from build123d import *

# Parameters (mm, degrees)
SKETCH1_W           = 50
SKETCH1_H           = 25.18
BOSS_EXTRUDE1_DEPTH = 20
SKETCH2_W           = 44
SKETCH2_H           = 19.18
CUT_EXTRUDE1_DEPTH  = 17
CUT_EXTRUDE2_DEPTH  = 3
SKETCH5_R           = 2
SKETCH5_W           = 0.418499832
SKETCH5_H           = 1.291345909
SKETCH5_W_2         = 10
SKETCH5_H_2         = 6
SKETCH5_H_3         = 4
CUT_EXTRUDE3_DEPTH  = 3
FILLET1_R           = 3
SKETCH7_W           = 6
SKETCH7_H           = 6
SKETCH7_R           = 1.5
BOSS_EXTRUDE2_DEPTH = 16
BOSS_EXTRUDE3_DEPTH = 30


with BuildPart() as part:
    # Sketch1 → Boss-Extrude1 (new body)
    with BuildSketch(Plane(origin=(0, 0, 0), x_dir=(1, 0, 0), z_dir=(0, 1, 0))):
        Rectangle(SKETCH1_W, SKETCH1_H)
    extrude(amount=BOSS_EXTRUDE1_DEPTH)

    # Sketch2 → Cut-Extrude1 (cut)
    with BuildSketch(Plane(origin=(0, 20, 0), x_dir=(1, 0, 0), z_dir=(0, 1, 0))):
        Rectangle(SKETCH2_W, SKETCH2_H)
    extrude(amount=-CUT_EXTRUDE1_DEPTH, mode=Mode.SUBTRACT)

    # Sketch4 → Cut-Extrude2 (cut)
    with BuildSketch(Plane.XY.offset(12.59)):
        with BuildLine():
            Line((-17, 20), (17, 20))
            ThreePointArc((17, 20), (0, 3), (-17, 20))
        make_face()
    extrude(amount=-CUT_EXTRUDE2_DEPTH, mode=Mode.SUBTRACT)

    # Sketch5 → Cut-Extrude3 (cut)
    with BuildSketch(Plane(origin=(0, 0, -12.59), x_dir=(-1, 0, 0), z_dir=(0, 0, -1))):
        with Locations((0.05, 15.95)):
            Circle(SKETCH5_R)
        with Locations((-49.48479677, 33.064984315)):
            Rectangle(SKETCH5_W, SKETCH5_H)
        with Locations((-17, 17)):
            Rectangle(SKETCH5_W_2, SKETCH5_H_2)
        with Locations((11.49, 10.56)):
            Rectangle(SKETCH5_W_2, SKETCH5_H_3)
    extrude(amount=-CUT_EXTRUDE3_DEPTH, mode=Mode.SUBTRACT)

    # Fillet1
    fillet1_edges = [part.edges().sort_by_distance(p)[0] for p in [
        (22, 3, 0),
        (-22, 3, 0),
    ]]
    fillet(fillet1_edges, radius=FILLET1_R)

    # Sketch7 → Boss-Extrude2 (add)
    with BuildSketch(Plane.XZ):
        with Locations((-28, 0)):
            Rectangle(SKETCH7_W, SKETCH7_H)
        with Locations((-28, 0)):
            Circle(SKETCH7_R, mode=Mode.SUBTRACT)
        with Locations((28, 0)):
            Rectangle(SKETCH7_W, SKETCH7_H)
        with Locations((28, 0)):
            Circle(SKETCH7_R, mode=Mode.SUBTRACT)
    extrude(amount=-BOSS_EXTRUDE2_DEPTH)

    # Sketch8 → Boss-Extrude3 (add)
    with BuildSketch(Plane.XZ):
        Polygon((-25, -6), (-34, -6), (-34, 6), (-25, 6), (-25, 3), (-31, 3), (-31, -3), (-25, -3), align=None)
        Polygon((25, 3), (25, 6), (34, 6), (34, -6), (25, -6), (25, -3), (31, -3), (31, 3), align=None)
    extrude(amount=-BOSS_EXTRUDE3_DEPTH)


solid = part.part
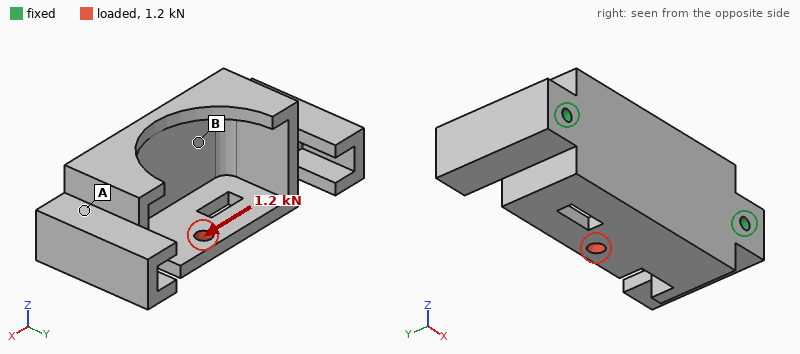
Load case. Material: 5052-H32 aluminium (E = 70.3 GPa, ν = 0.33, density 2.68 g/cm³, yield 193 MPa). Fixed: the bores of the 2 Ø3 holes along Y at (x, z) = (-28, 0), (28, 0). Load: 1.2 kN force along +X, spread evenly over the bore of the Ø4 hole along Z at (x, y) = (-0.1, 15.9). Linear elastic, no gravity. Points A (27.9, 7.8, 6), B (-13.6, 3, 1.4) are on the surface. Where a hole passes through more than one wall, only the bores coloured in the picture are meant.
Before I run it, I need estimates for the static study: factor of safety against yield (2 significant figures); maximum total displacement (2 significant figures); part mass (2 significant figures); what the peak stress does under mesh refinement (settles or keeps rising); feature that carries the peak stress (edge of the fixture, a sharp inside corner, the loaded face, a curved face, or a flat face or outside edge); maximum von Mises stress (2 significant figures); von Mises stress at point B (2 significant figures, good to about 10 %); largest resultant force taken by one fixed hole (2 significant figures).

3.3
17 µm
39 g
settles
the loaded face
59 MPa
6.8 MPa
720 N
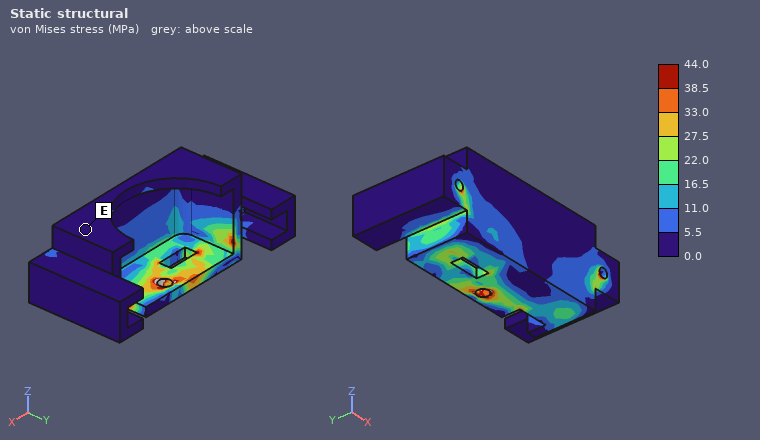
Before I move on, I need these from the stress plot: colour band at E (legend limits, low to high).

0.0 to 5.5 MPa
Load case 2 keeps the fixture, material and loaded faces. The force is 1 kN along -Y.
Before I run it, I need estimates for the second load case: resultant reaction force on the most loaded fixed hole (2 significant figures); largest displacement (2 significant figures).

510 N
31 µm
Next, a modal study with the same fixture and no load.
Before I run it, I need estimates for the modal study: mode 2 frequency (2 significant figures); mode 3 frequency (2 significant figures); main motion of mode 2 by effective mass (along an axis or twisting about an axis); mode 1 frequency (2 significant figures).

12 kHz
16 kHz
along Y
8800 Hz
